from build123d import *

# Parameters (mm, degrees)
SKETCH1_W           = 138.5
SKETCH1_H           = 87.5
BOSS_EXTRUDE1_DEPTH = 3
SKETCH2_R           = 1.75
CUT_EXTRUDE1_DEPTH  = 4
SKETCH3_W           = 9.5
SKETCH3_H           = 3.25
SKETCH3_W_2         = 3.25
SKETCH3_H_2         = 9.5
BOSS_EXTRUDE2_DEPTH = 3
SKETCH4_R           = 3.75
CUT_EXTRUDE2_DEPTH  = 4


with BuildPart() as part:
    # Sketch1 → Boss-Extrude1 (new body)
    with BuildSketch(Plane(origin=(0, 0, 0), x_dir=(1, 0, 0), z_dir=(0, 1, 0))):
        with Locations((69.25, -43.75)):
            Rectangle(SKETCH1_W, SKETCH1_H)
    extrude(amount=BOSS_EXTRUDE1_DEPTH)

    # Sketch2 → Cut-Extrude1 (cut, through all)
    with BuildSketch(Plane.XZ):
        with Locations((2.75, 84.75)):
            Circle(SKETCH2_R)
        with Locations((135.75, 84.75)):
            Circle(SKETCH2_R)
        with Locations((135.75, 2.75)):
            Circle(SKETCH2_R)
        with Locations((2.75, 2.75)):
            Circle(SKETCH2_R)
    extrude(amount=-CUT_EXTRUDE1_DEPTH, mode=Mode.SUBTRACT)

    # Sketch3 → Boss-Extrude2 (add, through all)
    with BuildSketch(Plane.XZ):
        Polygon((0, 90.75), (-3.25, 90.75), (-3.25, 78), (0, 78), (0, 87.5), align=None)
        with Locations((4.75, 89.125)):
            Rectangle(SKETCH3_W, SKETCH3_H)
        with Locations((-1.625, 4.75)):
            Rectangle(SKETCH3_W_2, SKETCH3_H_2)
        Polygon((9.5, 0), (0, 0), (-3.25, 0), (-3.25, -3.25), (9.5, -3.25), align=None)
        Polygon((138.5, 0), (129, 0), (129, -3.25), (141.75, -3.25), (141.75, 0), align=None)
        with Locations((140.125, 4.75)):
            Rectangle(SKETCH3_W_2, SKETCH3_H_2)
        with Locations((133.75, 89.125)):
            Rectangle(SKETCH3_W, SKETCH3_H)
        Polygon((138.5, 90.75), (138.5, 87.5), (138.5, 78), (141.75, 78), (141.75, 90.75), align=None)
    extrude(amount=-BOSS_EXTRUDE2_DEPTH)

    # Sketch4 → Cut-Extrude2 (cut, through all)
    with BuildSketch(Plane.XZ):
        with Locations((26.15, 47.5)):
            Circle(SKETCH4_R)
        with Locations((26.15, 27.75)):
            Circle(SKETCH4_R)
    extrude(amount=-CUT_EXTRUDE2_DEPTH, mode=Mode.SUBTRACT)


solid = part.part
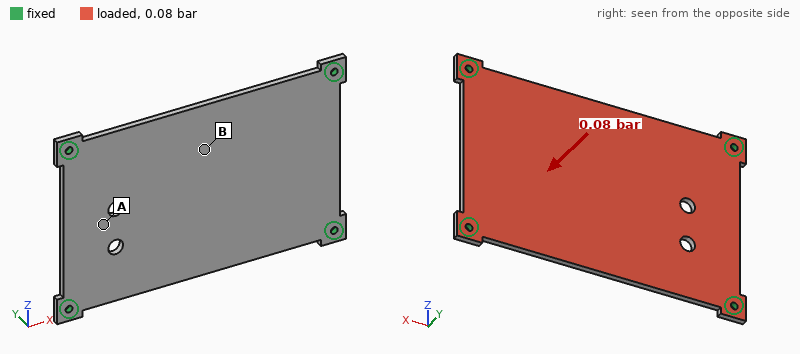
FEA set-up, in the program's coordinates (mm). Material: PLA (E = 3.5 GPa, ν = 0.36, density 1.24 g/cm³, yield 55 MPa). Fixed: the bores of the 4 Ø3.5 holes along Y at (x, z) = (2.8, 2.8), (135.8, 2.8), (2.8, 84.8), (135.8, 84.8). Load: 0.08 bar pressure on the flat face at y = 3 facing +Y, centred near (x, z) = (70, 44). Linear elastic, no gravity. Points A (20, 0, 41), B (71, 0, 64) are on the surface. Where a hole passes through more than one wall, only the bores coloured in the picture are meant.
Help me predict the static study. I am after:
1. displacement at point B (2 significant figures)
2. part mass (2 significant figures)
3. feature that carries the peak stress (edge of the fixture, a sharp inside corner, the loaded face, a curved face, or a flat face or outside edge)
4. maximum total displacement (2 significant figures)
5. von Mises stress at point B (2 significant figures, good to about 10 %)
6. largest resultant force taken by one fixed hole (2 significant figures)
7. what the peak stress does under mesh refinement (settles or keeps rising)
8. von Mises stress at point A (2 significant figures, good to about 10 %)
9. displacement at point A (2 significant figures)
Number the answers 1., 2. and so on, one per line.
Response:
1. 1.4 mm
2. 46 g
3. edge of the fixture
4. 1.4 mm
5. 4.8 MPa
6. 25 N
7. keeps rising
8. 2.3 MPa
9. 0.62 mm
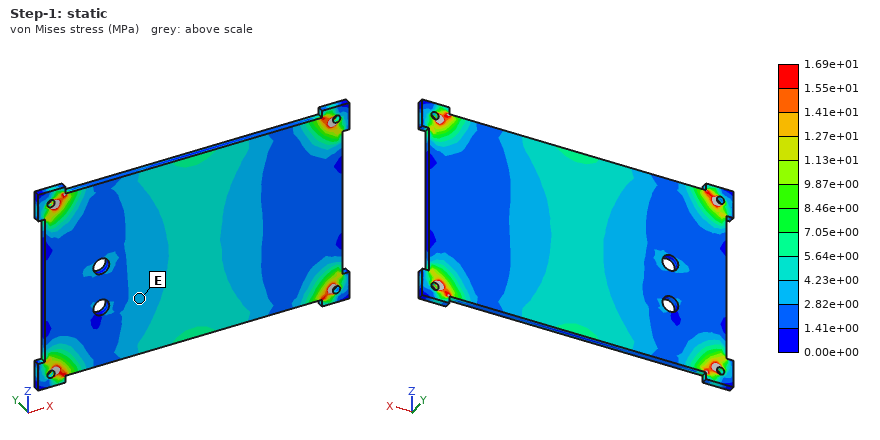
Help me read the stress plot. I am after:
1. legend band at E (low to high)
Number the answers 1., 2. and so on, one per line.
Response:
1. 2.82e+00 to 4.23e+00 MPa
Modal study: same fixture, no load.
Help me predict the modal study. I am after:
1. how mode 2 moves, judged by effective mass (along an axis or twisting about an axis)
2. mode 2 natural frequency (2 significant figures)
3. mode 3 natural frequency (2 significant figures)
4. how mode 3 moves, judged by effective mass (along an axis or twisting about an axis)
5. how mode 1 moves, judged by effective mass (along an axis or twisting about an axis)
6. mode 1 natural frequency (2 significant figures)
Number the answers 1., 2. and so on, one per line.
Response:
1. twisting about X
2. 400 Hz
3. 590 Hz
4. twisting about Z
5. along Y
6. 230 Hz
